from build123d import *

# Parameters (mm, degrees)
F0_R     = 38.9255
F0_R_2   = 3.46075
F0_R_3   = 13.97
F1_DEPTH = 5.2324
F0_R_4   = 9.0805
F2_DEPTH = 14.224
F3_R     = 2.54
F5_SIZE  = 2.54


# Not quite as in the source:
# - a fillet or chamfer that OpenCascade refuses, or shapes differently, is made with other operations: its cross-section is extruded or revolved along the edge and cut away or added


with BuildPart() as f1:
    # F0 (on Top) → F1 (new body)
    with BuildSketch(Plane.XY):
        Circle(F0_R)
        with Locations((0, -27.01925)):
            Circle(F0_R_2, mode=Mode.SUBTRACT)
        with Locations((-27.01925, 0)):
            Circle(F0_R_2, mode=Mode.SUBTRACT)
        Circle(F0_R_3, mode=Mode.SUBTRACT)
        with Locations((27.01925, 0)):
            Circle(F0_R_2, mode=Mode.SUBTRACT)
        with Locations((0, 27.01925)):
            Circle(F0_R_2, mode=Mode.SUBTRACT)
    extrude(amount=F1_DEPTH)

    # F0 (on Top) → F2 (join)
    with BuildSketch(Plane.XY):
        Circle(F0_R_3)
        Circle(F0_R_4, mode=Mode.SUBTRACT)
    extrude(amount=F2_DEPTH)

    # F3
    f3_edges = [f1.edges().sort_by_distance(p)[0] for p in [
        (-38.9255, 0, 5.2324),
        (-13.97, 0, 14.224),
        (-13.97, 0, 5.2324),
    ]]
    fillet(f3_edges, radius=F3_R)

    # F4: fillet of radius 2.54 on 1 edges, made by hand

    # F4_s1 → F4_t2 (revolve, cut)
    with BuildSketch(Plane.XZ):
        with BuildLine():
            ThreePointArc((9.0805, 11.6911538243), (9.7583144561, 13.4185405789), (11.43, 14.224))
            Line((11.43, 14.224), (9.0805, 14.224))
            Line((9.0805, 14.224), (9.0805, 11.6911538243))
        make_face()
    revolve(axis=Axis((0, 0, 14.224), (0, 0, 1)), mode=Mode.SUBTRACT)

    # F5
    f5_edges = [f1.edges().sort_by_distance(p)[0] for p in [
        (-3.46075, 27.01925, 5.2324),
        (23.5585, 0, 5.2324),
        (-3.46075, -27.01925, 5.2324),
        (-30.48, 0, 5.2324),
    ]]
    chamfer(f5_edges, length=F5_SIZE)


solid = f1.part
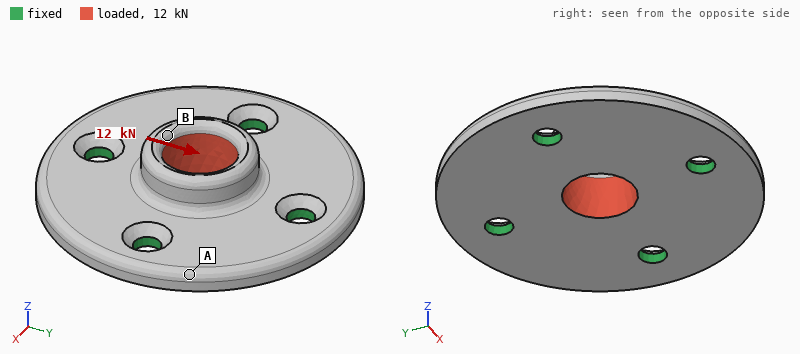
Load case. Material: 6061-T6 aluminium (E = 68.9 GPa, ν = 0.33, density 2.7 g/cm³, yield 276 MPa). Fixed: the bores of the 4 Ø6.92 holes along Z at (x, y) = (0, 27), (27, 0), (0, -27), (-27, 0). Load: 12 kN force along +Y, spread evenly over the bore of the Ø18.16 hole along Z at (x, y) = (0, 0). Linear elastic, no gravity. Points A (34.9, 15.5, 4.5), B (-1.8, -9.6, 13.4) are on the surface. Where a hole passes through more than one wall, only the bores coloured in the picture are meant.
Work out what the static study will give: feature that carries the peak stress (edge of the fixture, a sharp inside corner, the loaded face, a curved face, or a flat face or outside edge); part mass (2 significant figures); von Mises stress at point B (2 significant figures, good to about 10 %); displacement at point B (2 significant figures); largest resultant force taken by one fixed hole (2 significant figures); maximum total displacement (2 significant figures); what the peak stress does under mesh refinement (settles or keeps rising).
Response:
edge of the fixture
68 g
27 MPa
20 µm
4.1 kN
21 µm
keeps rising
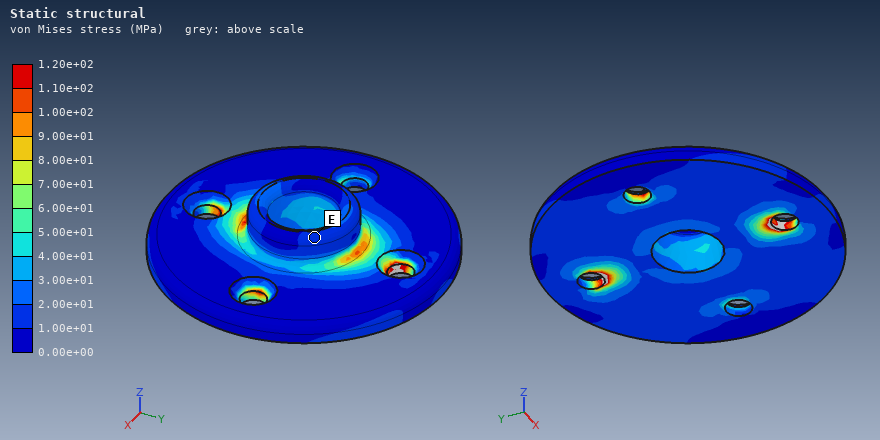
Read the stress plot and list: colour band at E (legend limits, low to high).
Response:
1.00e+01 to 2.00e+01 MPa
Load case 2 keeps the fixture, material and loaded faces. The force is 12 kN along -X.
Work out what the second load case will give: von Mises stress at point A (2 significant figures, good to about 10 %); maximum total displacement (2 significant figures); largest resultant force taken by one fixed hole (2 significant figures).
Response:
9.6 MPa
21 µm
4.1 kN
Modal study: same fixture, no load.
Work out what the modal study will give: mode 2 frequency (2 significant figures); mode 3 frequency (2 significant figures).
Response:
9800 Hz
9800 Hz
